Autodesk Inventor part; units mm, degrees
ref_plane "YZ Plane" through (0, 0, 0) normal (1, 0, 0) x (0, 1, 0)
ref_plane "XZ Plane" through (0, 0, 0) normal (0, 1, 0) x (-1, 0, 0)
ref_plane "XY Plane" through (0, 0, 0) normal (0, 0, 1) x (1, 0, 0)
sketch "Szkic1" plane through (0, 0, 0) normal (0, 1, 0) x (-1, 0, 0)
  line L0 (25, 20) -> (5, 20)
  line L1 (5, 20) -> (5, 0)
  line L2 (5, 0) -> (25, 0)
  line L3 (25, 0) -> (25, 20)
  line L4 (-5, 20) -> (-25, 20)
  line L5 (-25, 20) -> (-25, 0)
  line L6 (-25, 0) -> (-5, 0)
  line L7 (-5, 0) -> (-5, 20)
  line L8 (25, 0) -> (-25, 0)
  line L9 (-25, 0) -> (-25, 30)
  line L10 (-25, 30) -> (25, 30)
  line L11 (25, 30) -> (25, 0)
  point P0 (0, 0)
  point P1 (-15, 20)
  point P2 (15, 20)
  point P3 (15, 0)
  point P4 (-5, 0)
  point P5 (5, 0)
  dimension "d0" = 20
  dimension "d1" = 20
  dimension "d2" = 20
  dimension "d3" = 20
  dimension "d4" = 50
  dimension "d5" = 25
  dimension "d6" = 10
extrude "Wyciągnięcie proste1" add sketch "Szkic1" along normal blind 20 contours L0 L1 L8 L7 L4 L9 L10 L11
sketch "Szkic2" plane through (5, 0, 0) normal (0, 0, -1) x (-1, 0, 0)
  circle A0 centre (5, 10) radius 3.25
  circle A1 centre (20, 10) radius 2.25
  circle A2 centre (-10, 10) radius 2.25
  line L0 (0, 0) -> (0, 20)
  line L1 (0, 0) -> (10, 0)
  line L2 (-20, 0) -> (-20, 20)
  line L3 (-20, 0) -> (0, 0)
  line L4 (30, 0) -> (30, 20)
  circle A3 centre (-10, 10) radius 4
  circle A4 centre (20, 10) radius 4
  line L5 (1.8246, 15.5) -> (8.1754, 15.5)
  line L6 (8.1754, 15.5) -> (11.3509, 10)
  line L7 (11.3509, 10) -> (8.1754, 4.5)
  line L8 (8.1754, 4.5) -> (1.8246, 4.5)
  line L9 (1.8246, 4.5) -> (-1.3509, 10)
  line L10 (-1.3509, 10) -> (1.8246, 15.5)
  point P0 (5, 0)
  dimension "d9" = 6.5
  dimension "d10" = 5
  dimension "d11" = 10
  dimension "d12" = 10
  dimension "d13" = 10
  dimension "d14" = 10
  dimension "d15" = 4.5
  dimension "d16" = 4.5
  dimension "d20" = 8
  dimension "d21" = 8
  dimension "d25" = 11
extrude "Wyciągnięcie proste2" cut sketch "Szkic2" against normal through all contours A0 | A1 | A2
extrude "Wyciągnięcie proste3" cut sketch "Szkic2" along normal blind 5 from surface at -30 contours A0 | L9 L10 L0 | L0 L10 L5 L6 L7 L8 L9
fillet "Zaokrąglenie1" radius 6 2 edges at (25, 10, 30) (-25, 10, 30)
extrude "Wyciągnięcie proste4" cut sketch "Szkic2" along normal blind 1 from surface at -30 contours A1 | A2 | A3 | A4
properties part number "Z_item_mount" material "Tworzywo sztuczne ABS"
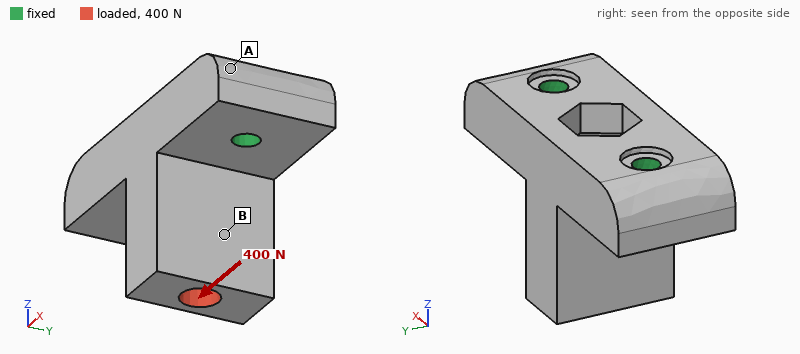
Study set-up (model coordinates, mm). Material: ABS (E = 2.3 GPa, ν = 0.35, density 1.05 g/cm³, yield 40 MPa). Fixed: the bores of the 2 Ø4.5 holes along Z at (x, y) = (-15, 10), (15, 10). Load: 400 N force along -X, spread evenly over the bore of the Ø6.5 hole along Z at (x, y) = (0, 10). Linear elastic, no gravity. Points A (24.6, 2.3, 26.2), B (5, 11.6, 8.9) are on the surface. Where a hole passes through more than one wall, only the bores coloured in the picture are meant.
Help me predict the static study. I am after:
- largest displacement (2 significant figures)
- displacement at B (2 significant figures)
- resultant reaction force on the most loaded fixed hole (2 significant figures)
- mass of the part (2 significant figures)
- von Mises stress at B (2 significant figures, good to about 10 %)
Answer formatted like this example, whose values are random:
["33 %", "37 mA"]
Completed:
["0.25 mm", "0.15 mm", "280 N", "13 g", "4.0 MPa"]
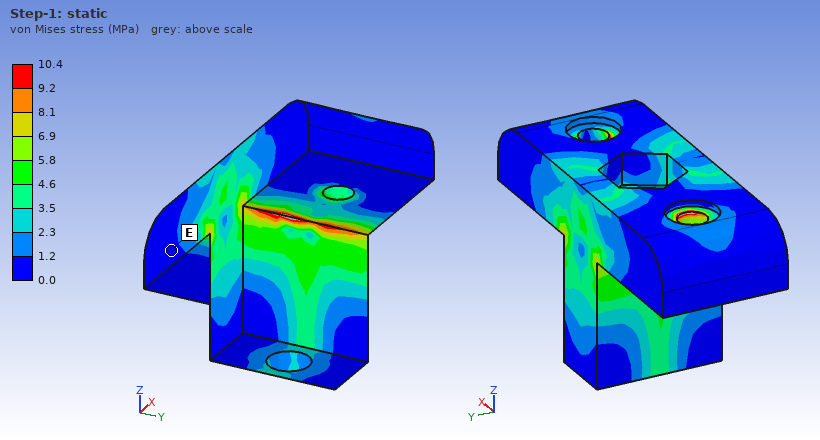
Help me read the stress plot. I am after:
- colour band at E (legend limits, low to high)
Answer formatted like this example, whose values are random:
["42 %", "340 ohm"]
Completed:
["0.0 to 1.2 MPa"]
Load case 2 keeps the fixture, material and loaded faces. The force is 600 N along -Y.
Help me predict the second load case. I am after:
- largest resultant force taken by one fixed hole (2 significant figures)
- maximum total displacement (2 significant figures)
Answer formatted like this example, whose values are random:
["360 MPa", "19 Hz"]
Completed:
["300 N", "0.47 mm"]
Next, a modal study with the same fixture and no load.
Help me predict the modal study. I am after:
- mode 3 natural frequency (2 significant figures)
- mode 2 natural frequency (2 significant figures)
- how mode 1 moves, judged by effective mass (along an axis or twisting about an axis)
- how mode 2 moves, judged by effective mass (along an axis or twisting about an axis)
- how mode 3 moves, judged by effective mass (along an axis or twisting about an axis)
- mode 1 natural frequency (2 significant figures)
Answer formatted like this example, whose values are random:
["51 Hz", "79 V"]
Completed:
["6700 Hz", "3800 Hz", "along Y", "along X", "along Z", "3100 Hz"]
